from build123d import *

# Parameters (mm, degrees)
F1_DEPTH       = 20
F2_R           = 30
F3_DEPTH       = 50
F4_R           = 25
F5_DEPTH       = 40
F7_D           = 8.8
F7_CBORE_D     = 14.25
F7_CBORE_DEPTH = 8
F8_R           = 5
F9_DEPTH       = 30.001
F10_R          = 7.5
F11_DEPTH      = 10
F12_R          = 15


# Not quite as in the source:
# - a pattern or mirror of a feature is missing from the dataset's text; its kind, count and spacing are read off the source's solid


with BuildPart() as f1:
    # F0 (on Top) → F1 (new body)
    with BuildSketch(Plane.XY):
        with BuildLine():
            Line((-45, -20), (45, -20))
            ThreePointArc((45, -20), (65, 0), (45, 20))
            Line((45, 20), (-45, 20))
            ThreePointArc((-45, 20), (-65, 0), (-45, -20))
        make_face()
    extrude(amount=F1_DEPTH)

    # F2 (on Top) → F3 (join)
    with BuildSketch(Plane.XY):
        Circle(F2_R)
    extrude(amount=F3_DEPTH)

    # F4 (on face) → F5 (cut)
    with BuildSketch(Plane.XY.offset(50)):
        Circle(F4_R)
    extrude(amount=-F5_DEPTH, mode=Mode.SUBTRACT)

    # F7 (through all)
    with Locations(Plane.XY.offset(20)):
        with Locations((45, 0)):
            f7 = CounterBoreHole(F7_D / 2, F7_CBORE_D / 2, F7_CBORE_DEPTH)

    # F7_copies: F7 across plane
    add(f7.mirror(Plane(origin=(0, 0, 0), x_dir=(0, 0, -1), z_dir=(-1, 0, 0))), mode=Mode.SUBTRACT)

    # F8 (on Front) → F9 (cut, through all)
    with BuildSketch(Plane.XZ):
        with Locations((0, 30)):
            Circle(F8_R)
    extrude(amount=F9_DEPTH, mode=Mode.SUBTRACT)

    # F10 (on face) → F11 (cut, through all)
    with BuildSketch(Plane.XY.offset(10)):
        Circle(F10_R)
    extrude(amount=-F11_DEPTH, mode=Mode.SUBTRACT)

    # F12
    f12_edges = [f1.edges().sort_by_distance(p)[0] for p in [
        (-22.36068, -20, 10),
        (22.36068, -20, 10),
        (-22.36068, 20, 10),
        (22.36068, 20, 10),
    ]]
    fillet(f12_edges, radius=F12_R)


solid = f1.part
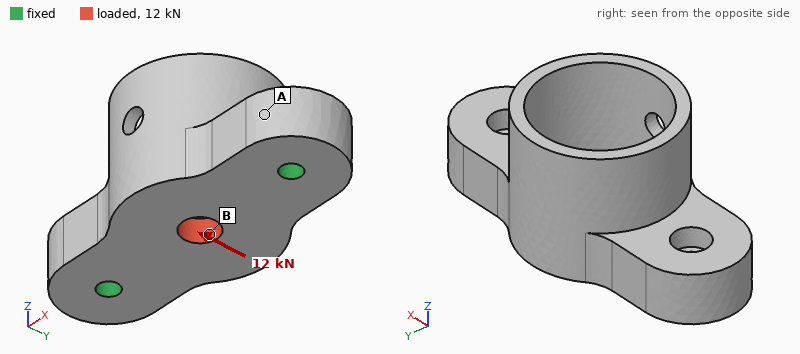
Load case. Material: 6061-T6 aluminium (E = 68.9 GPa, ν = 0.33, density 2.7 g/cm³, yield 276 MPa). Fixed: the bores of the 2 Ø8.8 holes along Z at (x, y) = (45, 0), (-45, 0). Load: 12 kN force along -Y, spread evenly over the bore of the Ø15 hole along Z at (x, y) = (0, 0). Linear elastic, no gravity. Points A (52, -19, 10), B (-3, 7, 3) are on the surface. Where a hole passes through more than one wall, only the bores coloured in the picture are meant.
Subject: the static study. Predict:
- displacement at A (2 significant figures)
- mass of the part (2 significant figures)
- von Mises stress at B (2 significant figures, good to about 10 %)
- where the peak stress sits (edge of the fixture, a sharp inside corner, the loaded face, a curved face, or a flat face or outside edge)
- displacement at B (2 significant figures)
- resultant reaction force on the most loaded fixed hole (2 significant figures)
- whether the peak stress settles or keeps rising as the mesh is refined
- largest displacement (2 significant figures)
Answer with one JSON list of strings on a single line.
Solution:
["8.0 µm", "300 g", "30 MPa", "edge of the fixture", "31 µm", "6.0 kN", "keeps rising", "32 µm"]
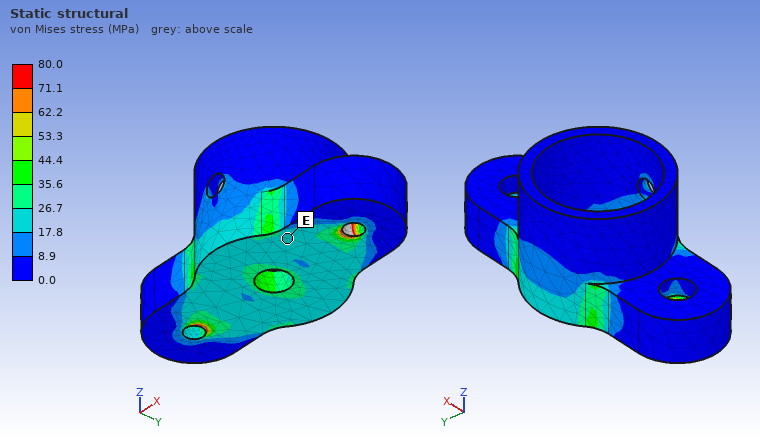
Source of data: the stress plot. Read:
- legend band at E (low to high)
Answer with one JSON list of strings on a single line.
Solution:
["17.8 to 26.7 MPa"]
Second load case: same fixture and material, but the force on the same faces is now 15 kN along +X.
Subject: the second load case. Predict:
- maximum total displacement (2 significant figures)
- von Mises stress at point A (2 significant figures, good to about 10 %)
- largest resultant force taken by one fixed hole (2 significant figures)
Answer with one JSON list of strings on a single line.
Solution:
["14 µm", "4.4 MPa", "7.5 kN"]
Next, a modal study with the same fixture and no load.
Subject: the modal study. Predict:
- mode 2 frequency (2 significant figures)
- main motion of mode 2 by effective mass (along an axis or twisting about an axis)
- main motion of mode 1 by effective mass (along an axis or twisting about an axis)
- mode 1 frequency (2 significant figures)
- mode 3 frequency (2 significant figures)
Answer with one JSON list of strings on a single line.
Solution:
["5200 Hz", "along Z", "along Y", "4100 Hz", "7000 Hz"]
